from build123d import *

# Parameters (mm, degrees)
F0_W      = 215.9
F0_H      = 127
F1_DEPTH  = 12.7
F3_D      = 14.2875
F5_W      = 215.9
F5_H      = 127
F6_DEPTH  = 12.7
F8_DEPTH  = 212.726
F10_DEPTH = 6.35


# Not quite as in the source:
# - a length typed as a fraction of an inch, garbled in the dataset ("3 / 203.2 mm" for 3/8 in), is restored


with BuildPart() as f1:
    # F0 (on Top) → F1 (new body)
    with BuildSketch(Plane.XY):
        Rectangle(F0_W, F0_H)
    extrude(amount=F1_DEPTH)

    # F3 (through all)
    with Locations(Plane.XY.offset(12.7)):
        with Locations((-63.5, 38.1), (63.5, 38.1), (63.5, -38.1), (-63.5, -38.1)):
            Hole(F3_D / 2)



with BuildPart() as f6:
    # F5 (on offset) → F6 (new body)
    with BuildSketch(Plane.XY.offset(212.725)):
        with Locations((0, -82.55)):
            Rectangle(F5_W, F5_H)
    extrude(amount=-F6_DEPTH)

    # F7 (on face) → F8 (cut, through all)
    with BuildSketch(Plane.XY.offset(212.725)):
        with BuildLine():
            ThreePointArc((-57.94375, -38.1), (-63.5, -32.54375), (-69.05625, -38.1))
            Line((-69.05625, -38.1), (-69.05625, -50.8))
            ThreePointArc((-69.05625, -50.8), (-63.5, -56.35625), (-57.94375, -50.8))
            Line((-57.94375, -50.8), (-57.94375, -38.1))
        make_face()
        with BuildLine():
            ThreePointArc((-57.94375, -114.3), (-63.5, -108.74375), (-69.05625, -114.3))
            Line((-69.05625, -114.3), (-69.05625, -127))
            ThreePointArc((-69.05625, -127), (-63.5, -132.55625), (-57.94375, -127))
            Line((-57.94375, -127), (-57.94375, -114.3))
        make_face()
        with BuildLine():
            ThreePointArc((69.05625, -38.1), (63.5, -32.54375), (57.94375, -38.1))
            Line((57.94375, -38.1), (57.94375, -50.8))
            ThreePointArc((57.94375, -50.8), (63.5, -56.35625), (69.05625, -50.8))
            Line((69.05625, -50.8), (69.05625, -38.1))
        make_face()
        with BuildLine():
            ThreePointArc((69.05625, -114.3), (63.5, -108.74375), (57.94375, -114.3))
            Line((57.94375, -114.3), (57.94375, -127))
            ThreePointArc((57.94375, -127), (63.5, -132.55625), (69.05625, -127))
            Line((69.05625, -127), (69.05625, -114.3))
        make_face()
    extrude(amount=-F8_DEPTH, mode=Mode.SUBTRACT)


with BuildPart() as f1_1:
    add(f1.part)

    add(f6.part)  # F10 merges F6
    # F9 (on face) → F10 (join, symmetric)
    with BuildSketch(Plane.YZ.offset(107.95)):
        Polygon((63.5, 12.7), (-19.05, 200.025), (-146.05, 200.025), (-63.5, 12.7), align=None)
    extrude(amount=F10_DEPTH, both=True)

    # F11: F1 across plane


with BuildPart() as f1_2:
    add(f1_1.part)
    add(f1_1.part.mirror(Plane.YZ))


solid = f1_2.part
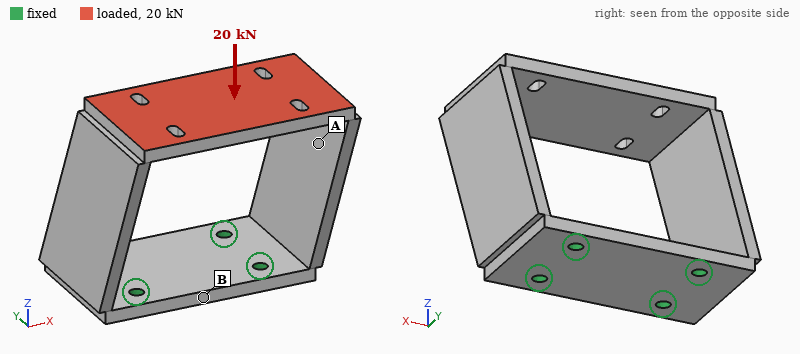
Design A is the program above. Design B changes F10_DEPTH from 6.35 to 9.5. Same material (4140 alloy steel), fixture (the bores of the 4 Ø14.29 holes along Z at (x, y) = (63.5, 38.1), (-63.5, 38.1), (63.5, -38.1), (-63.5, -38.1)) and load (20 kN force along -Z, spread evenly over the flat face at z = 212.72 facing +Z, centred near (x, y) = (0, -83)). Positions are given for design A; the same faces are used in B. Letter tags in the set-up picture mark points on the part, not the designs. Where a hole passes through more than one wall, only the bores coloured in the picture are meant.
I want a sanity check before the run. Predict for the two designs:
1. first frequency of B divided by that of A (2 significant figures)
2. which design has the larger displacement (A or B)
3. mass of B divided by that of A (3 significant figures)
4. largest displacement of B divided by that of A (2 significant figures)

1.2
A
1.23
0.69
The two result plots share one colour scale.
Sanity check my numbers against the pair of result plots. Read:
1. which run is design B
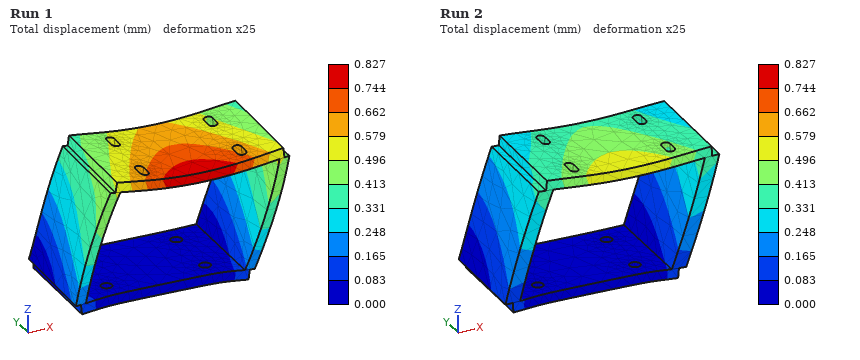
Run 2
